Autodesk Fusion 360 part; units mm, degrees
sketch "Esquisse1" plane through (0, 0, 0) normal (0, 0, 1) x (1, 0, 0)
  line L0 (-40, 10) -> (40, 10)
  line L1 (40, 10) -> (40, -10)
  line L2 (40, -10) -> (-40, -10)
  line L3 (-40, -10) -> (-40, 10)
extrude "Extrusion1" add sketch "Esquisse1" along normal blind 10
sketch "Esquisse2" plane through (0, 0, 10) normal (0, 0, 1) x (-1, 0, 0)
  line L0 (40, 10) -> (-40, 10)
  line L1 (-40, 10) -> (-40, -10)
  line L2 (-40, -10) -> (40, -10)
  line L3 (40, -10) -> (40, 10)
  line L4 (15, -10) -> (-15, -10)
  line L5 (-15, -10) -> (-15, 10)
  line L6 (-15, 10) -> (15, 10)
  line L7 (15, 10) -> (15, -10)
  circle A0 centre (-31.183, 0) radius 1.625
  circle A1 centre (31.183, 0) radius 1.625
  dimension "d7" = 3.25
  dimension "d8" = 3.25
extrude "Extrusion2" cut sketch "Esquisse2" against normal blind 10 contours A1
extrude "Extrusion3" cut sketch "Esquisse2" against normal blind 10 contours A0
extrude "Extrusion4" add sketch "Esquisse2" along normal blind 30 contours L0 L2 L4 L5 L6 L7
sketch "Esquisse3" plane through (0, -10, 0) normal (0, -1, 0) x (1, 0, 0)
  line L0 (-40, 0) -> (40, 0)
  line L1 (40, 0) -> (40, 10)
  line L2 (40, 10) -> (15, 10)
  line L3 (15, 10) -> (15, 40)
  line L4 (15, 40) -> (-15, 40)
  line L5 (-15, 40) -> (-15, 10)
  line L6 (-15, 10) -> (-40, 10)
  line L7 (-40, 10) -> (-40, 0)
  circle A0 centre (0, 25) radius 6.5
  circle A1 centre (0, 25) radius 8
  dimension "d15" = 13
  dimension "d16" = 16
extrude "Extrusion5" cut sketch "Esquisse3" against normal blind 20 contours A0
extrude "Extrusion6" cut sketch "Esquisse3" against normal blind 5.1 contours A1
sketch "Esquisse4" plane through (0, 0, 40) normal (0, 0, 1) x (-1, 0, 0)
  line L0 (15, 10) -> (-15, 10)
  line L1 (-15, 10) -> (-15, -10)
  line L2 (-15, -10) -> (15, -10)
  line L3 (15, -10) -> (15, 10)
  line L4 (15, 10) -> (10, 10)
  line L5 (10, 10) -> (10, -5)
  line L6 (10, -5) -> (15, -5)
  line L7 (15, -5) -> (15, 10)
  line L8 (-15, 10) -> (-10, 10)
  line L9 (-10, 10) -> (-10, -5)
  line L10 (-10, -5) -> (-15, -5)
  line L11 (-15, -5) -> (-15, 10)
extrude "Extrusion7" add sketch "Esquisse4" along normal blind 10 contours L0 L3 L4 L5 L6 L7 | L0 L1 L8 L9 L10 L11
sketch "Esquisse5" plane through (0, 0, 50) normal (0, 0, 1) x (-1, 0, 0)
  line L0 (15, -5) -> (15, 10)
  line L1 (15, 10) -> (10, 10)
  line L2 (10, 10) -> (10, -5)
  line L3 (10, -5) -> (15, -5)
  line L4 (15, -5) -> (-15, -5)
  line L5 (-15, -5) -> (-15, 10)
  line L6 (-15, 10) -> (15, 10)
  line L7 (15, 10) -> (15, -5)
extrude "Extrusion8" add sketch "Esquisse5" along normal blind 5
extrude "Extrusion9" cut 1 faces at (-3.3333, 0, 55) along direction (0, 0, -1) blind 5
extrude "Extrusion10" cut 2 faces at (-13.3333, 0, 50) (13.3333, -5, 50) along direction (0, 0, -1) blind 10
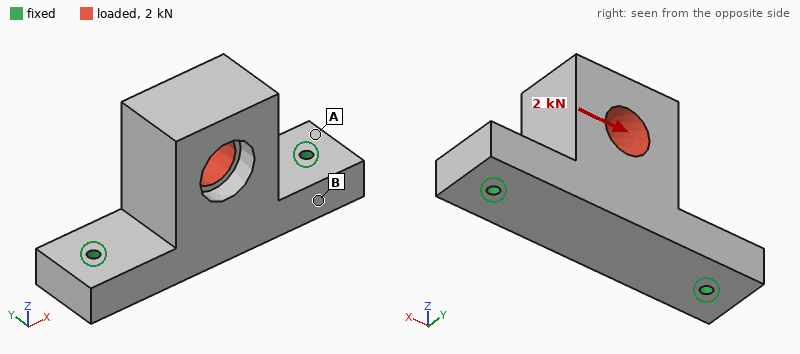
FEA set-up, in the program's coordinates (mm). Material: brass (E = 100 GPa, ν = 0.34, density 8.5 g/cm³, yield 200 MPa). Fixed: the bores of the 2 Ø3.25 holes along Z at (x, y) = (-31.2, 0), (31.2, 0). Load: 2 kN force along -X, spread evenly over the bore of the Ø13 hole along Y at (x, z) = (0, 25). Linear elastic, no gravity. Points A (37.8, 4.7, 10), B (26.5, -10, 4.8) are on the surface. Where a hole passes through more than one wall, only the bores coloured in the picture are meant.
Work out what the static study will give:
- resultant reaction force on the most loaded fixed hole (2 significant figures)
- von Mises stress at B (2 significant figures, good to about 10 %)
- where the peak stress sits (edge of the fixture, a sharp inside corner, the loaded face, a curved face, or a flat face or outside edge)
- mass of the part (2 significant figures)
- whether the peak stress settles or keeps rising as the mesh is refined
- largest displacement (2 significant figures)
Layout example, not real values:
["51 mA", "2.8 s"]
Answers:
["1.3 kN", "7.7 MPa", "edge of the fixture", "260 g", "keeps rising", "18 µm"]
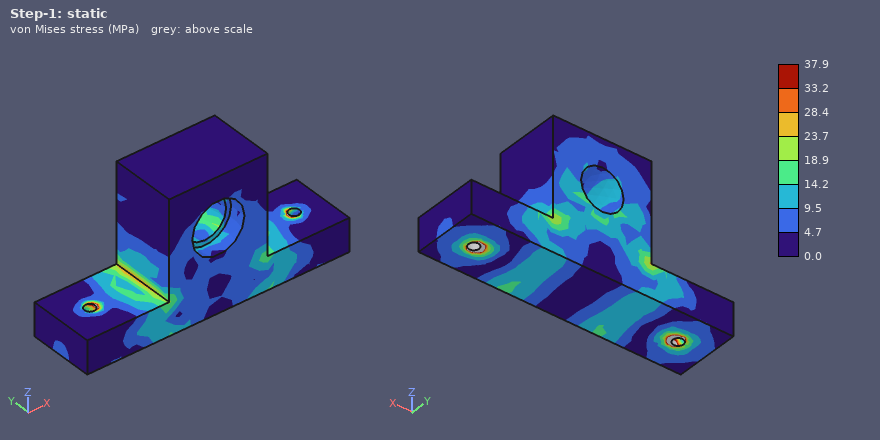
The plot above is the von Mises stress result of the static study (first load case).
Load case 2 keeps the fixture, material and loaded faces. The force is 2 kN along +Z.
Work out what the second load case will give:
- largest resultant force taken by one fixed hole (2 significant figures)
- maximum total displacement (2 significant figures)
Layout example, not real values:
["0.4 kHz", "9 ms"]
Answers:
["1.1 kN", "18 µm"]
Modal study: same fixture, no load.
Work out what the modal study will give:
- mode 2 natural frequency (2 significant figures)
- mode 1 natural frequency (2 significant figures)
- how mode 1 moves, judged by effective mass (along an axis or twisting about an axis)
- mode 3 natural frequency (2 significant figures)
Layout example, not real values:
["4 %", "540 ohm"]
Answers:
["5200 Hz", "2300 Hz", "along Y", "5400 Hz"]
